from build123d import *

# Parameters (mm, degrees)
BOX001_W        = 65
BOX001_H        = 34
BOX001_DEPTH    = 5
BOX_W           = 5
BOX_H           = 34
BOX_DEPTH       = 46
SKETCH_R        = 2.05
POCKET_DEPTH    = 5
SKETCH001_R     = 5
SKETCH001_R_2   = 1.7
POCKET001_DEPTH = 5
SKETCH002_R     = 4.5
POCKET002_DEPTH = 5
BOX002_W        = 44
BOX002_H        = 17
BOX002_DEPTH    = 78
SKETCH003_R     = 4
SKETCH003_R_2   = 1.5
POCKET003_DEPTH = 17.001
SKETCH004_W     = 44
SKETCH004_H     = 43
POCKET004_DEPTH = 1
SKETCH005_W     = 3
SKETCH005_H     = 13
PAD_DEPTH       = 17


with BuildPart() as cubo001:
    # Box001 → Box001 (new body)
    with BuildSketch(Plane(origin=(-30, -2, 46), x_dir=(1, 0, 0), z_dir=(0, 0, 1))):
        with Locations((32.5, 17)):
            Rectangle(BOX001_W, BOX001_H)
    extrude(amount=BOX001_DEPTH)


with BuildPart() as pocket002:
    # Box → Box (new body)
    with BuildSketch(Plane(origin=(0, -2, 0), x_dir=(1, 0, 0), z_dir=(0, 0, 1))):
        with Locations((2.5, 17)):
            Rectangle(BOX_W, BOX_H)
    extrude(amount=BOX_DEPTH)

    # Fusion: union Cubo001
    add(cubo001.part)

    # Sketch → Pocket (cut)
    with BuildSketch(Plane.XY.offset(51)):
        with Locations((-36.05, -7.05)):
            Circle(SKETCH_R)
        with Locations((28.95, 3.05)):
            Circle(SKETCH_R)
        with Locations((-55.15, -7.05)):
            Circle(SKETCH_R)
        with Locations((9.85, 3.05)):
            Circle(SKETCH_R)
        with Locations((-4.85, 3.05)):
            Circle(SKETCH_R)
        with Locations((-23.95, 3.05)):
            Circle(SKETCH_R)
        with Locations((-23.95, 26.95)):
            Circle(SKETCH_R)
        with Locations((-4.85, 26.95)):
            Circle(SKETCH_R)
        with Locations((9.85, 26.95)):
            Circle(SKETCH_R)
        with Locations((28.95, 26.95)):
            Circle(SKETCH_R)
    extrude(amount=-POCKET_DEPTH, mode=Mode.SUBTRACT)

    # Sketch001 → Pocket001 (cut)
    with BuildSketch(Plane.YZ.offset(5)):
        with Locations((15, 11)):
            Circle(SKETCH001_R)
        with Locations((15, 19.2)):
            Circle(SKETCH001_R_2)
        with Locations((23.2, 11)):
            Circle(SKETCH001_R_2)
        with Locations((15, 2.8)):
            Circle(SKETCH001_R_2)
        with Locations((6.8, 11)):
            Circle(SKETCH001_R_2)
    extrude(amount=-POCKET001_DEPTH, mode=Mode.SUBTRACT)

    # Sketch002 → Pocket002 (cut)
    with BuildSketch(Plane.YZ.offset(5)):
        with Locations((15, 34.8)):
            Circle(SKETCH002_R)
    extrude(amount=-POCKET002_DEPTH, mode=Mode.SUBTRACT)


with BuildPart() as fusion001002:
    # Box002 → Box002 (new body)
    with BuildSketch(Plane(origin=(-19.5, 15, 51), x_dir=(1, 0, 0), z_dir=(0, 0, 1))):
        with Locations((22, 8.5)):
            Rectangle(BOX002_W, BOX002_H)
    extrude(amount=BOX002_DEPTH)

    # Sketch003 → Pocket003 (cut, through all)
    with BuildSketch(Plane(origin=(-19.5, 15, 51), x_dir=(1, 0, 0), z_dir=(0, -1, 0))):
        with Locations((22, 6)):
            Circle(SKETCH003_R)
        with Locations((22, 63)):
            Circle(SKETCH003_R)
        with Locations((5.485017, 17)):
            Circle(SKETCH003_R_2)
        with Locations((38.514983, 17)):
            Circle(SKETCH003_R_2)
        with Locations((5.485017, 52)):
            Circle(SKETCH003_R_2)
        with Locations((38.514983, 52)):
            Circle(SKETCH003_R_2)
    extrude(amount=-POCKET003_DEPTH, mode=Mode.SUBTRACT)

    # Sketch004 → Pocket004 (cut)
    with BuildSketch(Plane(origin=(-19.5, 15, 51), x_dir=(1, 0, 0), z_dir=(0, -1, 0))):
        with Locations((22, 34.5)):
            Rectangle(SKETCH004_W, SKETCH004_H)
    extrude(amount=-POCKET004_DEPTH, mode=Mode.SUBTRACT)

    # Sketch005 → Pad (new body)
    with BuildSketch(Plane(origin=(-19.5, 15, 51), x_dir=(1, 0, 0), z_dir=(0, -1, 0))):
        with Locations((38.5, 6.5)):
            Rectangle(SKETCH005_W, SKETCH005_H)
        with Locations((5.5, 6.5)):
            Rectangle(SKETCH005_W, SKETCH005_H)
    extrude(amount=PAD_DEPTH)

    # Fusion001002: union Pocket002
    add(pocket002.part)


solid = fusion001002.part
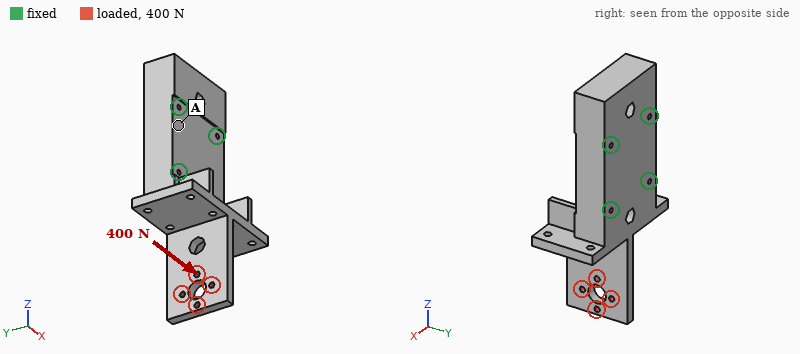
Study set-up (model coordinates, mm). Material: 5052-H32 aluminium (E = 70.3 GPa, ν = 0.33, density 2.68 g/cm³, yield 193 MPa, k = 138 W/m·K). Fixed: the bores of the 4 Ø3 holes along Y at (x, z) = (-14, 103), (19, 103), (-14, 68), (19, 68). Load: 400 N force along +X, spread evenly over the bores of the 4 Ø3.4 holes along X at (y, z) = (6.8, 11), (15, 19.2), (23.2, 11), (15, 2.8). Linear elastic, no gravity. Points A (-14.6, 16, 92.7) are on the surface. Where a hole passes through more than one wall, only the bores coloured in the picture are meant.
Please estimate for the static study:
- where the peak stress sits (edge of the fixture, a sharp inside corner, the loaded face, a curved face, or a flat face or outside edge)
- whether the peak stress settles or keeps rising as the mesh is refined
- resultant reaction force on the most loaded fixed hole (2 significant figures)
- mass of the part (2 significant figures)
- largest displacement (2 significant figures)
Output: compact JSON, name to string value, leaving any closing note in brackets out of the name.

{"where the peak stress sits": "a sharp inside corner", "whether the peak stress settles or keeps rising as the mesh is refined": "keeps rising", "resultant reaction force on the most loaded fixed hole": "650 N", "mass of the part": "200 g", "largest displacement": "0.46 mm"}
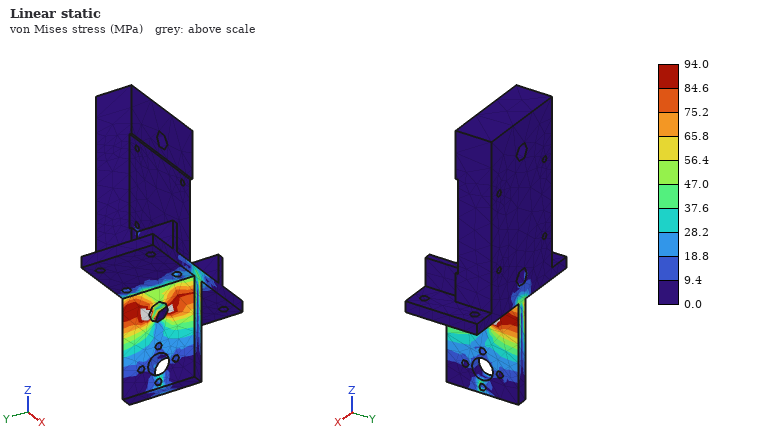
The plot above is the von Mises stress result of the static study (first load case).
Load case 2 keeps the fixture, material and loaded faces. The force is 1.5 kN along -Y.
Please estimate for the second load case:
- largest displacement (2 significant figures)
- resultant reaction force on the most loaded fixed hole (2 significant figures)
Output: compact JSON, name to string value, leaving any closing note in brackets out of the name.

{"largest displacement": "0.25 mm", "resultant reaction force on the most loaded fixed hole": "1.2 kN"}
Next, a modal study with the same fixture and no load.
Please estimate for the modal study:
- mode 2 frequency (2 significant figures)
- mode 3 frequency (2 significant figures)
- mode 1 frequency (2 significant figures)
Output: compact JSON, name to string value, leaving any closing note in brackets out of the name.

{"mode 2 frequency": "3900 Hz", "mode 3 frequency": "5000 Hz", "mode 1 frequency": "1800 Hz"}
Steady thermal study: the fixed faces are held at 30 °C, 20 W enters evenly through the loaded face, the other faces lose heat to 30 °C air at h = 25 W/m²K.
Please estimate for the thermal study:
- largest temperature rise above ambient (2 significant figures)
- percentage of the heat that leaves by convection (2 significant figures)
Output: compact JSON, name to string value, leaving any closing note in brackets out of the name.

{"largest temperature rise above ambient": "44 K", "percentage of the heat that leaves by convection": "16 %"}
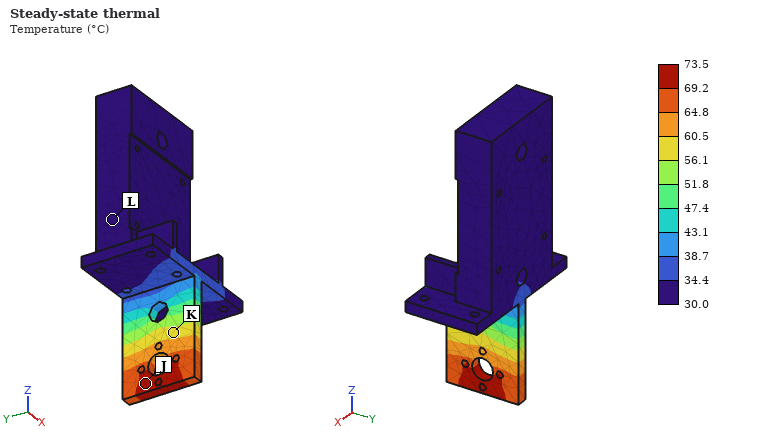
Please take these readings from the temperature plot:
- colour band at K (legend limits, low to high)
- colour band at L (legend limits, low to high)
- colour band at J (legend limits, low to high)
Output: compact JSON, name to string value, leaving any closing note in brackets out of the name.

{"colour band at K": "56.1 to 60.5 °C", "colour band at L": "30.0 to 34.4 °C", "colour band at J": "69.2 to 73.5 °C"}
